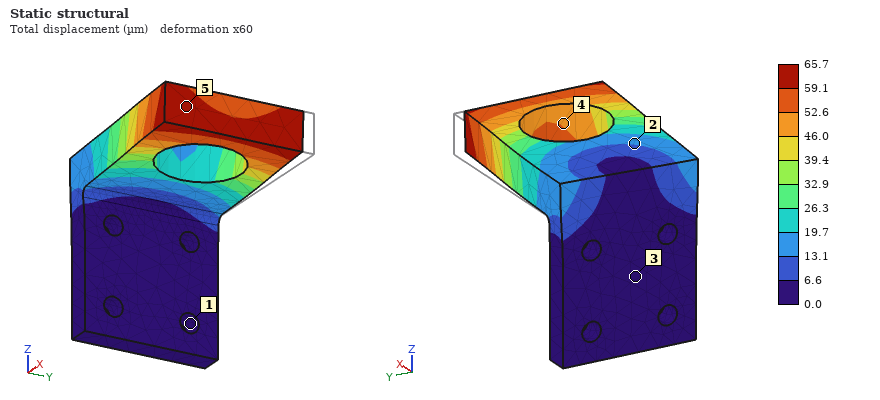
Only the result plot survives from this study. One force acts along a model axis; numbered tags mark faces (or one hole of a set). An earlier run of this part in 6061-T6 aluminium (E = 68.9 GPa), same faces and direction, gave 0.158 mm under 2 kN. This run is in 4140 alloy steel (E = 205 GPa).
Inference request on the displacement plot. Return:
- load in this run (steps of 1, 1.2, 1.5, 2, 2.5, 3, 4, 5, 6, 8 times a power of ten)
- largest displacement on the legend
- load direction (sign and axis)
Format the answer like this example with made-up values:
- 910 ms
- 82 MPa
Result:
- 2.5 kN
- 65.7 µm
- -Y
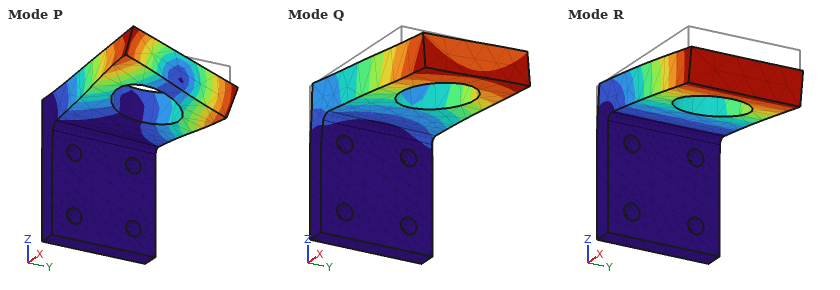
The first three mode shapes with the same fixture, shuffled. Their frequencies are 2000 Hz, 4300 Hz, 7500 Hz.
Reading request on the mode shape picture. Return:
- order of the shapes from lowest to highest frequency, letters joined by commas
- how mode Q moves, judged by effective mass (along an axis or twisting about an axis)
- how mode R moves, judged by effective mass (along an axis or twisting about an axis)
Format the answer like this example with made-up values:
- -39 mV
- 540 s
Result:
- R, Q, P
- along Y
- along Z
